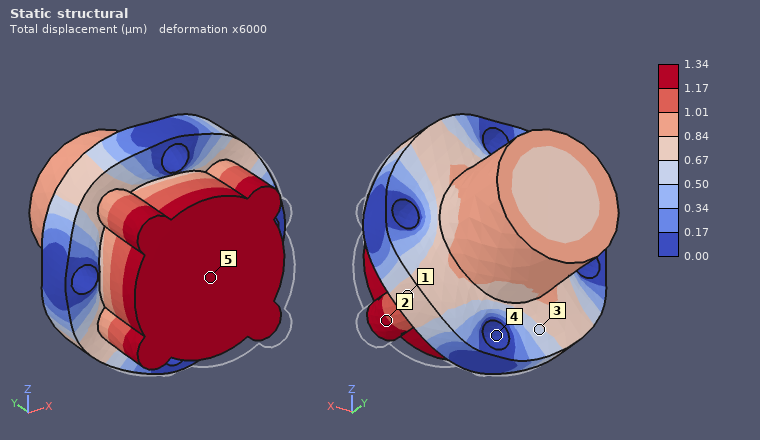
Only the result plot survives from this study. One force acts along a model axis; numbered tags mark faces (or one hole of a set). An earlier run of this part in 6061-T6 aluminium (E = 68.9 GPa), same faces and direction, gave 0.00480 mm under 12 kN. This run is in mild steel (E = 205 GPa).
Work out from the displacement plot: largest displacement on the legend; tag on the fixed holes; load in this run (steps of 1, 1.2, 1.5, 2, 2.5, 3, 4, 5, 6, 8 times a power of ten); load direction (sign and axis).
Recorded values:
1.34 µm
4
10 kN
+Y
